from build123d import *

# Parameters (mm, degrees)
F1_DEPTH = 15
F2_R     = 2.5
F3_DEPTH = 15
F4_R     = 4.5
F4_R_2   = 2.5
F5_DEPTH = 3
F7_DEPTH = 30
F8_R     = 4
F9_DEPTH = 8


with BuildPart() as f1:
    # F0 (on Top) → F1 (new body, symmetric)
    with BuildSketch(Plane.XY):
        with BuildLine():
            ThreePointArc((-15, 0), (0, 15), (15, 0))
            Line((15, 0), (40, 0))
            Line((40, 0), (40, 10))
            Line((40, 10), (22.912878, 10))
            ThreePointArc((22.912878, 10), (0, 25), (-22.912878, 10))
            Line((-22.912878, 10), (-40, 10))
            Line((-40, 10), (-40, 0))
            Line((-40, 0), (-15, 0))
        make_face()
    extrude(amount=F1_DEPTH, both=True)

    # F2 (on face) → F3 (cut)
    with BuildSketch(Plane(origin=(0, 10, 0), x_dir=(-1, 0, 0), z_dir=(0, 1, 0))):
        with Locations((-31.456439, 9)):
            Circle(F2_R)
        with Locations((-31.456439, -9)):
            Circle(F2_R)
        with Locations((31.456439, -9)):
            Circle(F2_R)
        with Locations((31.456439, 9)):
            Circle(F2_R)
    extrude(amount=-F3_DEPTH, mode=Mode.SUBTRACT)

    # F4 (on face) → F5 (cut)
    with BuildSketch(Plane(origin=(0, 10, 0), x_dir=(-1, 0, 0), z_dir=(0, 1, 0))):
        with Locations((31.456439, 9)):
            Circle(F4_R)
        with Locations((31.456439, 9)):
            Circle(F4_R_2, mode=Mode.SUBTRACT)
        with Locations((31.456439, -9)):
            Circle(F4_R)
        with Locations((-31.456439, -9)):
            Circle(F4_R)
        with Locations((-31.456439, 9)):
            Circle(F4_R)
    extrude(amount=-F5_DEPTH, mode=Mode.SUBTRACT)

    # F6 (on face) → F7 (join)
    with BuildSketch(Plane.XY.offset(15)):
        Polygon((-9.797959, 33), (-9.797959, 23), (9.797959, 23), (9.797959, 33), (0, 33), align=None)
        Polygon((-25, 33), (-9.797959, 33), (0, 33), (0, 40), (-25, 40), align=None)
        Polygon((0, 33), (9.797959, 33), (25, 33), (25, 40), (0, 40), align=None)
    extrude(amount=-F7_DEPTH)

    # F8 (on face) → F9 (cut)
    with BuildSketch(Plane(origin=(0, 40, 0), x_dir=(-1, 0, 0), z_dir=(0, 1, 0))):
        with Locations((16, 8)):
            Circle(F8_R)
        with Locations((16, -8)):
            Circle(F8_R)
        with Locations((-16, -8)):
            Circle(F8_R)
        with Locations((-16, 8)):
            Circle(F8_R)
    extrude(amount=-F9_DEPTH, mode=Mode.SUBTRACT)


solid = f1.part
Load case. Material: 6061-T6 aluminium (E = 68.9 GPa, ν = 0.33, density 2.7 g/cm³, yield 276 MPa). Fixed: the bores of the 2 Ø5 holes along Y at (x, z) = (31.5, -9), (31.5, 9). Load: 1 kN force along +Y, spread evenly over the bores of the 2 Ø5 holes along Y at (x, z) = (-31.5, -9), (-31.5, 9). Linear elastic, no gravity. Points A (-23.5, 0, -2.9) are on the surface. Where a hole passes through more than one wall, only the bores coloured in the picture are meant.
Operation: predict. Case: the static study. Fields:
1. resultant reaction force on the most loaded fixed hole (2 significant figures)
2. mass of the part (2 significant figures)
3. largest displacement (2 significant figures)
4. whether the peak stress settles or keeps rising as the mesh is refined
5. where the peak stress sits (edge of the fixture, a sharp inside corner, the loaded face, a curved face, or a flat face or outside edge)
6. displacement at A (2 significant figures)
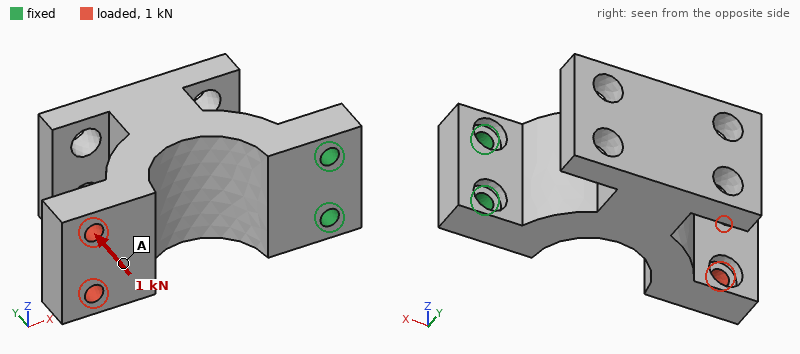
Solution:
500 N
110 g
0.75 mm
keeps rising
edge of the fixture
0.53 mm
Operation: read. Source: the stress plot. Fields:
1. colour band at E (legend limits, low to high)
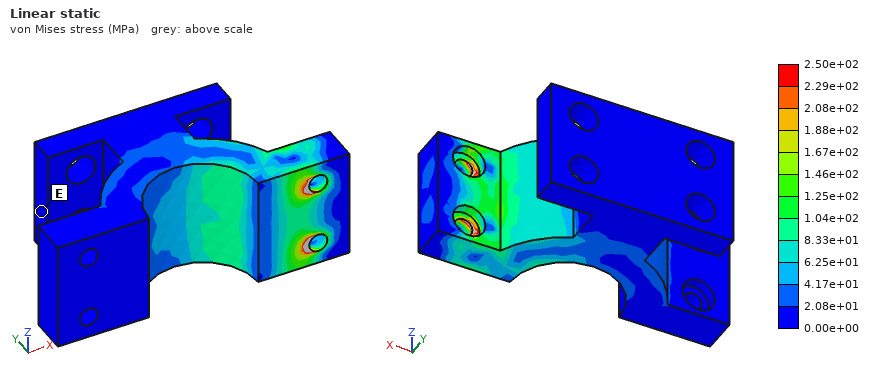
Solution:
0.00e+00 to 2.08e+01 MPa
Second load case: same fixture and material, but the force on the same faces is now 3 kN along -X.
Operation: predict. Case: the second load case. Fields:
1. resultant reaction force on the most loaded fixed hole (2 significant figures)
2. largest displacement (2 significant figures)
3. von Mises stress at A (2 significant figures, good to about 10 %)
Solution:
1.5 kN
0.37 mm
16 MPa
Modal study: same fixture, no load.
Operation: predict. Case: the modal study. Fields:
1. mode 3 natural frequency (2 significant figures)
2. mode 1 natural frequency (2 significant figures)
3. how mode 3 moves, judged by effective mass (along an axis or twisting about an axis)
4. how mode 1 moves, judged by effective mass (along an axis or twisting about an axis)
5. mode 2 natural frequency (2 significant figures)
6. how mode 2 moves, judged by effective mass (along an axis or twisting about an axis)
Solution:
3400 Hz
1000 Hz
along Z
along Y
2500 Hz
along Z
